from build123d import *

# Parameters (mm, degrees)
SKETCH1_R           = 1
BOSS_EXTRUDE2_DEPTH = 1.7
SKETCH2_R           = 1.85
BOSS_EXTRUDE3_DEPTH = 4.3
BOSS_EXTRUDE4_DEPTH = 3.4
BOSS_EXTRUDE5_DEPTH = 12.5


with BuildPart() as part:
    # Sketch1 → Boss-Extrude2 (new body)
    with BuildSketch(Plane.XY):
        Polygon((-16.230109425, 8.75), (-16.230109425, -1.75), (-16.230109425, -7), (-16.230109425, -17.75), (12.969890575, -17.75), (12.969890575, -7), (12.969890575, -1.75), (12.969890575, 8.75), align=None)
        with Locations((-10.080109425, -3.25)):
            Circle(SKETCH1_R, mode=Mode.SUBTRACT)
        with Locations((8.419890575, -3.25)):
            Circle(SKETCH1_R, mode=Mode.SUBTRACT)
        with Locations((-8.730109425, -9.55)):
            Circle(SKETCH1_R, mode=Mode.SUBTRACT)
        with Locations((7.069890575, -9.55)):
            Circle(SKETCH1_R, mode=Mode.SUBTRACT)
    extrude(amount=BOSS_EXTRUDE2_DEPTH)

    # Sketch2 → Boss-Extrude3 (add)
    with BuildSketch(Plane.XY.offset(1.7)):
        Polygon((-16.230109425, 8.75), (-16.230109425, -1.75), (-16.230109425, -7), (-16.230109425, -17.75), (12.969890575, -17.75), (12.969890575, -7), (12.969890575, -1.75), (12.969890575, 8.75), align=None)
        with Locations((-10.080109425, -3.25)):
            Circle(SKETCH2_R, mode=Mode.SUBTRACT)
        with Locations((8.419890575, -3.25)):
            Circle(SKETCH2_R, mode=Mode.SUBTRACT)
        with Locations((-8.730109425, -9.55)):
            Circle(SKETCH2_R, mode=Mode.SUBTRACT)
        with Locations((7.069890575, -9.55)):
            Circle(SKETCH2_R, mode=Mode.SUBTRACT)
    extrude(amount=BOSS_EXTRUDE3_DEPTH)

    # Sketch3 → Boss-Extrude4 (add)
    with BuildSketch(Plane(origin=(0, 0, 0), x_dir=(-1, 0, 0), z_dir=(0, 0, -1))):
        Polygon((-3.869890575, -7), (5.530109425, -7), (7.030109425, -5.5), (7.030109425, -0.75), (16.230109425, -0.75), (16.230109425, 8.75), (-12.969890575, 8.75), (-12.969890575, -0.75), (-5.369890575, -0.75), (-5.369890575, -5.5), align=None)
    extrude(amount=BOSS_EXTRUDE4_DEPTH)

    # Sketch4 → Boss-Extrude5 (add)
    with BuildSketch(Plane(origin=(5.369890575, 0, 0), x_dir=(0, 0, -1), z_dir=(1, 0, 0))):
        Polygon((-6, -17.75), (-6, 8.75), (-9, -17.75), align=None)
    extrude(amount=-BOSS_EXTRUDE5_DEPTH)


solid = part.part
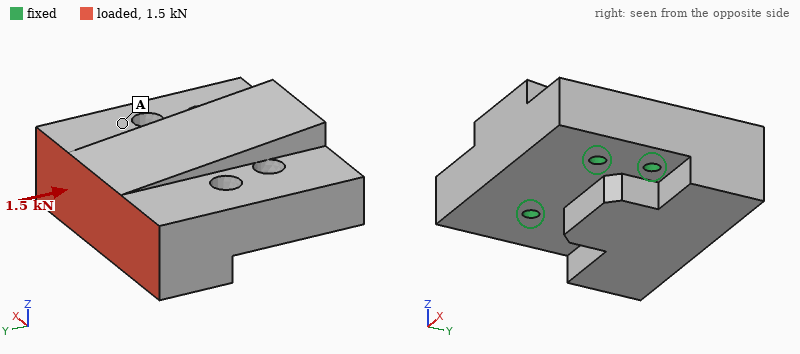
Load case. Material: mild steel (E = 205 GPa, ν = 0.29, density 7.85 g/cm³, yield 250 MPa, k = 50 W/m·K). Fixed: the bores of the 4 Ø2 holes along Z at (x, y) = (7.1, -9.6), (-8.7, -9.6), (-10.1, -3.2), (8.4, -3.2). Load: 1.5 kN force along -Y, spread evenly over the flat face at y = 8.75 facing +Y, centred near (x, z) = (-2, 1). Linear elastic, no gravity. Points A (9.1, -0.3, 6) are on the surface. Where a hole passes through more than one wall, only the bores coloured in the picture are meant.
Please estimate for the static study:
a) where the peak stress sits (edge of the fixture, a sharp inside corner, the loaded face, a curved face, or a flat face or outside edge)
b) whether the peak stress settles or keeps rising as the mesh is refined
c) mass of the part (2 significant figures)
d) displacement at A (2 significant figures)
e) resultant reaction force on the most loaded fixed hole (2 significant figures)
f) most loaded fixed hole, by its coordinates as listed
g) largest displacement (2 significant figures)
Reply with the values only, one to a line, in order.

edge of the fixture
keeps rising
48 g
0.56 µm
520 N
(-10.1, -3.2)
1.1 µm
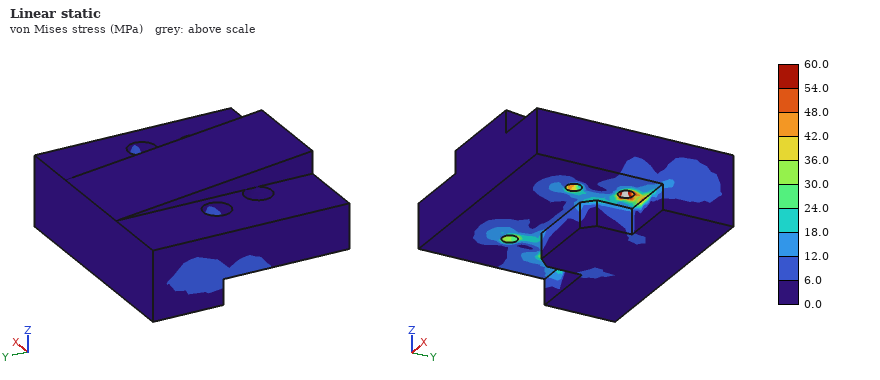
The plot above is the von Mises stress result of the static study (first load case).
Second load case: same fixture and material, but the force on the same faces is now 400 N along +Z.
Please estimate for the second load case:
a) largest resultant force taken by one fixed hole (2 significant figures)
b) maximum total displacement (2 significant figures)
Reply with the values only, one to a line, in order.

510 N
6.2 µm
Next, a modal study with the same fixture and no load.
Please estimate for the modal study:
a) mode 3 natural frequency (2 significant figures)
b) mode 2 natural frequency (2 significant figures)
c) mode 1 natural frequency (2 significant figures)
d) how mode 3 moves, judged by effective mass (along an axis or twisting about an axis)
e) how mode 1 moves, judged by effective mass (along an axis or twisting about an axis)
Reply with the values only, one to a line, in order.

27 kHz
26 kHz
12 kHz
along Z
along Z
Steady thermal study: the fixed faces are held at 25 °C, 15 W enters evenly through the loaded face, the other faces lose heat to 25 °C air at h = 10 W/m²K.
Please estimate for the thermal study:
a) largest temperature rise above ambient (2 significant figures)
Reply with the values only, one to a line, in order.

24 K
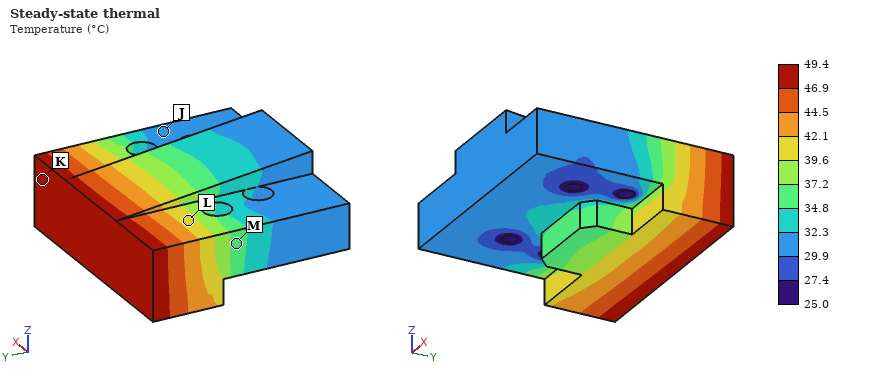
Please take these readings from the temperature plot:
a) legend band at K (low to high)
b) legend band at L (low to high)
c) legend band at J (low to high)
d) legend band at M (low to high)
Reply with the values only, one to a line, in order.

46.9 to 49.4 °C
39.6 to 42.1 °C
29.9 to 32.3 °C
34.8 to 37.2 °C
